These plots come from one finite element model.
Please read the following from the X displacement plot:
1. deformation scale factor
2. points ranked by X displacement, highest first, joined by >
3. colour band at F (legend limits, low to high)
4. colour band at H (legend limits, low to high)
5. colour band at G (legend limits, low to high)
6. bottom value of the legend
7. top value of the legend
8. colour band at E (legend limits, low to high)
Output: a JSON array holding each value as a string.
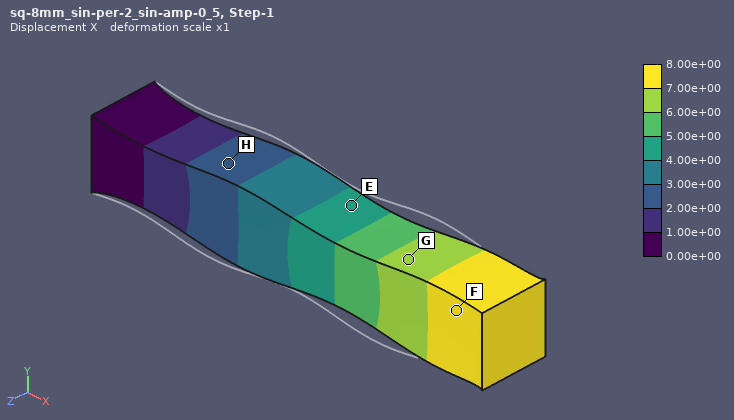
["1", "F > G > E > H", "7.00e+00 to 8.00e+00", "2.00e+00 to 3.00e+00", "6.00e+00 to 7.00e+00", "0.00e+00", "8.00e+00", "4.00e+00 to 5.00e+00"]
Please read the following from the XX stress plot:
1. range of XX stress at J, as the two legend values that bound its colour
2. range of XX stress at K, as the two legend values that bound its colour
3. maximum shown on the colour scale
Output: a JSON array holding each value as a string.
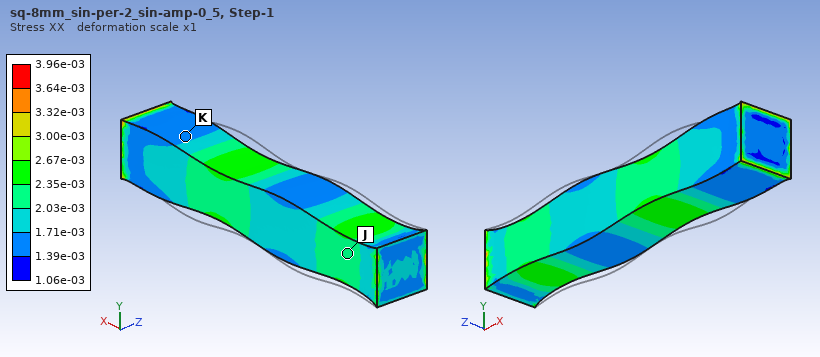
["2.03e-03 to 2.35e-03", "1.39e-03 to 1.71e-03", "3.96e-03"]
